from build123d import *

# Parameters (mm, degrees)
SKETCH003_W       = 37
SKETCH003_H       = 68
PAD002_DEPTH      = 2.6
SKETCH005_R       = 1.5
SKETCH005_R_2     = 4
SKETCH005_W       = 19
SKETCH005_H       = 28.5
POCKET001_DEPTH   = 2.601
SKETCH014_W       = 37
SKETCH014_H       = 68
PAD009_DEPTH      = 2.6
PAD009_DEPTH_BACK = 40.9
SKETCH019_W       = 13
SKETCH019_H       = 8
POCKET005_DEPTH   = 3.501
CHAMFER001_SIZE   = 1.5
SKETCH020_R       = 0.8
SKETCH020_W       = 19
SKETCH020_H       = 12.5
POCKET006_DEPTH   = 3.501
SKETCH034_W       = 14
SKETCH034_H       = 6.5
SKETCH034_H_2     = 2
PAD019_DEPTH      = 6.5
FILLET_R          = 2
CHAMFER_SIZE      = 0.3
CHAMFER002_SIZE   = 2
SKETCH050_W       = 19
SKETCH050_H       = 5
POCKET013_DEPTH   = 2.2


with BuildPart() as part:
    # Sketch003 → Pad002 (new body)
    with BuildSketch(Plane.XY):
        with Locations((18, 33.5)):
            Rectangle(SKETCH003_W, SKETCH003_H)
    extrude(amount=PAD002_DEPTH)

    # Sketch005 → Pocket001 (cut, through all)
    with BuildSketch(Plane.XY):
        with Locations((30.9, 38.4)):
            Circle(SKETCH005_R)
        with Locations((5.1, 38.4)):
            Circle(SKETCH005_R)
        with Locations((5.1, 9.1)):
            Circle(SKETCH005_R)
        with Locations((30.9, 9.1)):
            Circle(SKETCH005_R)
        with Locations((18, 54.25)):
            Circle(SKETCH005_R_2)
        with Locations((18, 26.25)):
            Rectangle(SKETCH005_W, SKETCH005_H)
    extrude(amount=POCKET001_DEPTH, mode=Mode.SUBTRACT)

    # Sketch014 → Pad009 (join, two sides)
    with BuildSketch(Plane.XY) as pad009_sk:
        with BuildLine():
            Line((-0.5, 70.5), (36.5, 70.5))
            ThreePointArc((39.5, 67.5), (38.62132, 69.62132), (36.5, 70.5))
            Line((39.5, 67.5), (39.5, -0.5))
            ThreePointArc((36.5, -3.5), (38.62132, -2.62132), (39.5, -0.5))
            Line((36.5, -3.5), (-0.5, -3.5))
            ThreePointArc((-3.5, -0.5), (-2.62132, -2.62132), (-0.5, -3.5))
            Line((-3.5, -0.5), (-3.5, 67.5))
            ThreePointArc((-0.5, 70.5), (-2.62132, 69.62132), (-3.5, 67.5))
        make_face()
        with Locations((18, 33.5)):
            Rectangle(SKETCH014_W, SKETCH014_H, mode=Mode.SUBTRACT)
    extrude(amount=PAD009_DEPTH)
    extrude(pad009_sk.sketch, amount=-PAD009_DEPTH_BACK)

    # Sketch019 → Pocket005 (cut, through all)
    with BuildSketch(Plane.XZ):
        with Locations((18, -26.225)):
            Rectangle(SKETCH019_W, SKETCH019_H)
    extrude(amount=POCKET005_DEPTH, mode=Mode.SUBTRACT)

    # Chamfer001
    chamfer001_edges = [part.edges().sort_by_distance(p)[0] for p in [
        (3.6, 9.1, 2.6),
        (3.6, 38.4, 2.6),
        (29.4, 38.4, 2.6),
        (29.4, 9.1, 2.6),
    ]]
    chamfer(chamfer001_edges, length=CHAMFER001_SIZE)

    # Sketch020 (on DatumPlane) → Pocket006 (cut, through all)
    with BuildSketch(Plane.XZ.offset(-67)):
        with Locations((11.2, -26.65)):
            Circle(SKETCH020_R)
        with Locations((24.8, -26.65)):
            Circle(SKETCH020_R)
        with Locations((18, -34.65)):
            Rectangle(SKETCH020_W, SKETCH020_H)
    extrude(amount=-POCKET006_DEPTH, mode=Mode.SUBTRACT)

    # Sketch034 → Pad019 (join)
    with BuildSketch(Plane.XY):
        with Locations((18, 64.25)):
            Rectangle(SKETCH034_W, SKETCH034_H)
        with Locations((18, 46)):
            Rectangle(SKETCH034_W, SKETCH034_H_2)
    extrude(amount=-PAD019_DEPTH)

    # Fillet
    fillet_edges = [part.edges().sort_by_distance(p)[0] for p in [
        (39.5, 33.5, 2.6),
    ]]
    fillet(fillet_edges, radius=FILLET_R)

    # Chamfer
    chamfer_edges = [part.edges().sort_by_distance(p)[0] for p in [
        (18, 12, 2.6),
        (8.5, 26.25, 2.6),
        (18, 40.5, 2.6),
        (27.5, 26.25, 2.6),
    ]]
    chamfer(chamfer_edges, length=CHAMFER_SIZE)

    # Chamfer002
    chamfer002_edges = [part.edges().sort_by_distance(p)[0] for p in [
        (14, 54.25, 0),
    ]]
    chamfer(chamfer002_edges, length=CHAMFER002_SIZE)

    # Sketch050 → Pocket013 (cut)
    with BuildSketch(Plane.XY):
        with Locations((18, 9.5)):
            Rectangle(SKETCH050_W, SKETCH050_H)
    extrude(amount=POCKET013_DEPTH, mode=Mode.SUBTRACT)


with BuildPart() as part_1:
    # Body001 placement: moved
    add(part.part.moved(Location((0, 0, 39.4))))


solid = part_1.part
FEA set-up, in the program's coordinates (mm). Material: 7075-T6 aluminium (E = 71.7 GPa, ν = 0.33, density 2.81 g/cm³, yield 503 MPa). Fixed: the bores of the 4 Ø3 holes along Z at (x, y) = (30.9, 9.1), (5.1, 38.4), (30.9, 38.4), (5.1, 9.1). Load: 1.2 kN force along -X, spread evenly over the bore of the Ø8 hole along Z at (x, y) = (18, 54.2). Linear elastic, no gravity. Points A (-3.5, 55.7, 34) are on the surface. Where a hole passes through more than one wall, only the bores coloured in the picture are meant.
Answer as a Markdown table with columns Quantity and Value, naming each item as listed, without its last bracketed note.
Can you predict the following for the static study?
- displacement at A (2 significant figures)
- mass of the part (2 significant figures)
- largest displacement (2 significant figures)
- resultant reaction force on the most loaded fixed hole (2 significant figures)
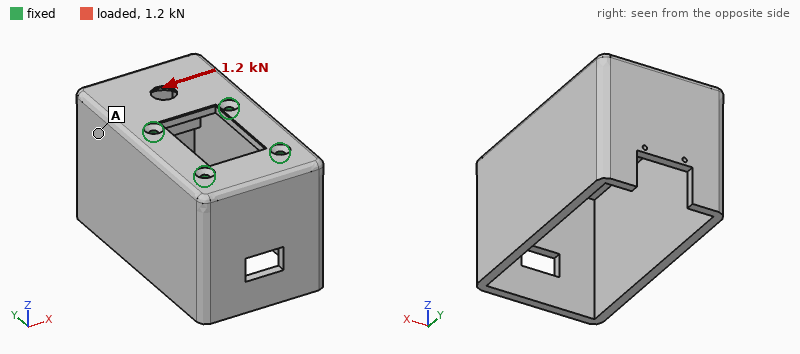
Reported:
| Quantity | Value |
|---|---|
| displacement at A | 14 µm |
| mass of the part | 92 g |
| largest displacement | 20 µm |
| resultant reaction force on the most loaded fixed hole | 740 N |
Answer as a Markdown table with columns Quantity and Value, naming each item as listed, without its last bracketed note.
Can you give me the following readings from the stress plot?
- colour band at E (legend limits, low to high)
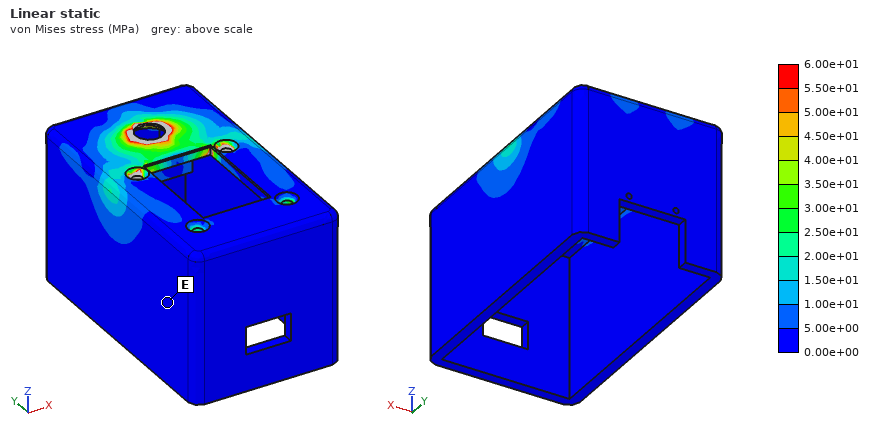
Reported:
| Quantity | Value |
|---|---|
| colour band at E | 0.00e+00 to 5.00e+00 MPa |
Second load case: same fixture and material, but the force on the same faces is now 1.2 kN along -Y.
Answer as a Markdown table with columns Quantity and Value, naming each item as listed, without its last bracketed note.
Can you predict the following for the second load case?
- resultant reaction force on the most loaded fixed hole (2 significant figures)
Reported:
| Quantity | Value |
|---|---|
| resultant reaction force on the most loaded fixed hole | 540 N |
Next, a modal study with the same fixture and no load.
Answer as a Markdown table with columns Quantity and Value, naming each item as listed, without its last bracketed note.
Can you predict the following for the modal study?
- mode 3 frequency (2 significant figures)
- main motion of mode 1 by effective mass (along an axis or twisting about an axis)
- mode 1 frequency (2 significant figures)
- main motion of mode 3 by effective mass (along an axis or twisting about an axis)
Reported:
| Quantity | Value |
|---|---|
| mode 3 frequency | 2300 Hz |
| main motion of mode 1 by effective mass | along X |
| mode 1 frequency | 1700 Hz |
| main motion of mode 3 by effective mass | along X |
